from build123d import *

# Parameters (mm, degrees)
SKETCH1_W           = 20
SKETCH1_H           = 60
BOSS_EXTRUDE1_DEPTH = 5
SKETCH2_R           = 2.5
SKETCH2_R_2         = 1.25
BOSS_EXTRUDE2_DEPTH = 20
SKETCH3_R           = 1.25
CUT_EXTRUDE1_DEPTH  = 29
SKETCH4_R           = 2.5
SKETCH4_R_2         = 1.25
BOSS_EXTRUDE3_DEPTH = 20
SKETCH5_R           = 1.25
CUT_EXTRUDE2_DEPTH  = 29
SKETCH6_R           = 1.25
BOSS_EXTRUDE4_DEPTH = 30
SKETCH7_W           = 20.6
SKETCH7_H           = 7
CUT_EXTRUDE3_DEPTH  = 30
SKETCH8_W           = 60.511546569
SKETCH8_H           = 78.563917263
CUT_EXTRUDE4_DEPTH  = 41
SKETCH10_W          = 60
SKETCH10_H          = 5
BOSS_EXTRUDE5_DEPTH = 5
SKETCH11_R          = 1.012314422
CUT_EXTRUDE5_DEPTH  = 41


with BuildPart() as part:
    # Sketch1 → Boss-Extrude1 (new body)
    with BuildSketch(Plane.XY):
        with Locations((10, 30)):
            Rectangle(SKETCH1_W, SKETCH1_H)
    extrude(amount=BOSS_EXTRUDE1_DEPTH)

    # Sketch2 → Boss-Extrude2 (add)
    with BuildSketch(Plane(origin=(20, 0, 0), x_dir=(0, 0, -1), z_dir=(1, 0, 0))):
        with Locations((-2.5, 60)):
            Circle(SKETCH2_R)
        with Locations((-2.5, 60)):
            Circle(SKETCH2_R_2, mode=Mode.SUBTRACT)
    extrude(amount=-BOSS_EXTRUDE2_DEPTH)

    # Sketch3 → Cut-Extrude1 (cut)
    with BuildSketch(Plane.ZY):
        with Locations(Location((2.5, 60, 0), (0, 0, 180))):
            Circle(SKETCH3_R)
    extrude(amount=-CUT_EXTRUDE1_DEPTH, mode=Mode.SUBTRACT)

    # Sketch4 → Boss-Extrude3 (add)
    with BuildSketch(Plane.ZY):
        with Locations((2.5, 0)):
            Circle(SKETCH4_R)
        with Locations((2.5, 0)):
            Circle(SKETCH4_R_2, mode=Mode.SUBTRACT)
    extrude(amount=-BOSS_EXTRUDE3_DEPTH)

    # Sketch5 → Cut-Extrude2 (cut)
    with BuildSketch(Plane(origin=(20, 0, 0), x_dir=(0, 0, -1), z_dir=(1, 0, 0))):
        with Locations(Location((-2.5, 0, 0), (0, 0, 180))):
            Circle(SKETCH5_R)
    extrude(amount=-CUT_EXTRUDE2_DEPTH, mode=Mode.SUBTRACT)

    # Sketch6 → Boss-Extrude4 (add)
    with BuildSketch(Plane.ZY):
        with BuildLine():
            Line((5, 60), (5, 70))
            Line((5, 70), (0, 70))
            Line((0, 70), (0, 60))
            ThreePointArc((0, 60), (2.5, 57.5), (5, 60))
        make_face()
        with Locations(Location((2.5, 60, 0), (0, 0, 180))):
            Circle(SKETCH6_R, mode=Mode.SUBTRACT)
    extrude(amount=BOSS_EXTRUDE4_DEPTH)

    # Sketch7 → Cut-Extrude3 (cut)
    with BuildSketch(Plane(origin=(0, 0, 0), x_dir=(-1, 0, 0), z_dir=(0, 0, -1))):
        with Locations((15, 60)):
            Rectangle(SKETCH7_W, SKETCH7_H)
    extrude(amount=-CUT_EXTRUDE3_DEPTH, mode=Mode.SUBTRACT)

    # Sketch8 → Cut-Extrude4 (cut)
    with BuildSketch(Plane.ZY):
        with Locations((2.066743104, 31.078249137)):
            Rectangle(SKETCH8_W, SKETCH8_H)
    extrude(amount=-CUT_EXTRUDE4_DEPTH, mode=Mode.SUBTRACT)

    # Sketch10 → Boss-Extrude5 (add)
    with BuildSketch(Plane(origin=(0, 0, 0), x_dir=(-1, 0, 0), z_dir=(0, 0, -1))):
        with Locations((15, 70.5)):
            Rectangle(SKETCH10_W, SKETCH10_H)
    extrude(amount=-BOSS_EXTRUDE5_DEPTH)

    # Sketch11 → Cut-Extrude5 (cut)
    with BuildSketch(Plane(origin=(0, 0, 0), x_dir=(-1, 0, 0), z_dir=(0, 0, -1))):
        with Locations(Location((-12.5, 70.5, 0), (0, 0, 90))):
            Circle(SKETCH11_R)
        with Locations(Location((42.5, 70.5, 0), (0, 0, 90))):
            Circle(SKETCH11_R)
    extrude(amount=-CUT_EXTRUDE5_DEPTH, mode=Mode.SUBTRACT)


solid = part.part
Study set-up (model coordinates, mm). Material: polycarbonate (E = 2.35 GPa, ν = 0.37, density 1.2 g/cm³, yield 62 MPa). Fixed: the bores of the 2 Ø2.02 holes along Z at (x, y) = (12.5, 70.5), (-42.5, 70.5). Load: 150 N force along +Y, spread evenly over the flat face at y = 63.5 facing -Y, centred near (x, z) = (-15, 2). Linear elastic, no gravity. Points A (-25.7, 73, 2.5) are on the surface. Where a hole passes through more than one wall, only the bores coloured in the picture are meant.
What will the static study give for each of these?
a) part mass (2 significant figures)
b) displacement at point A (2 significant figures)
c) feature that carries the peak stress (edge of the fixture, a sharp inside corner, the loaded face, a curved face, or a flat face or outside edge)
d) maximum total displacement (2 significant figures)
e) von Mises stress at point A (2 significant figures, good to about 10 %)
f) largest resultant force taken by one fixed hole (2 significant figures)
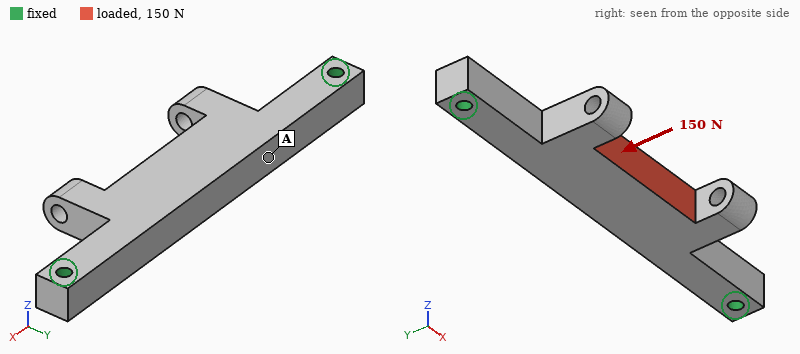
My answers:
2.8 g
0.35 mm
edge of the fixture
0.42 mm
8.6 MPa
110 N
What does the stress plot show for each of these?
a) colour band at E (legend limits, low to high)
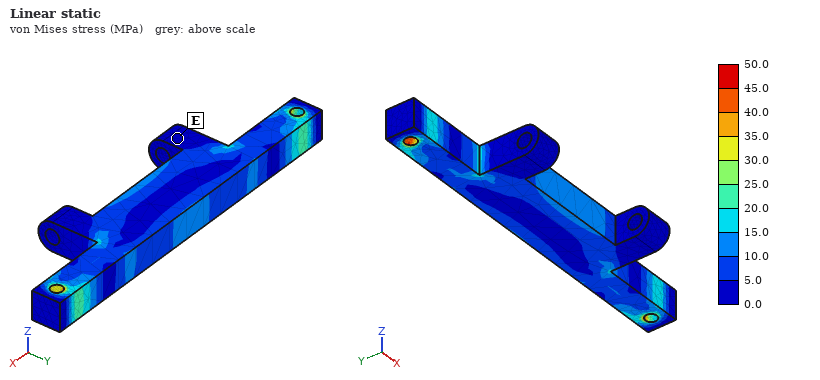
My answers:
0.0 to 5.0 MPa
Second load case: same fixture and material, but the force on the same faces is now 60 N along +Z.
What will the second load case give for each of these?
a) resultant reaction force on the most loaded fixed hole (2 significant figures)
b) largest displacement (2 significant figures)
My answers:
30 N
0.73 mm
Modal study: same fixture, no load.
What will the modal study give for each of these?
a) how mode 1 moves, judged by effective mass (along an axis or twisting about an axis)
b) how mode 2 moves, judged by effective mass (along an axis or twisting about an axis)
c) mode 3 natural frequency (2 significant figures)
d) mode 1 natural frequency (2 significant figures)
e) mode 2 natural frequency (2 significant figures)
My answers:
along Z
along Y
3200 Hz
1600 Hz
2300 Hz
